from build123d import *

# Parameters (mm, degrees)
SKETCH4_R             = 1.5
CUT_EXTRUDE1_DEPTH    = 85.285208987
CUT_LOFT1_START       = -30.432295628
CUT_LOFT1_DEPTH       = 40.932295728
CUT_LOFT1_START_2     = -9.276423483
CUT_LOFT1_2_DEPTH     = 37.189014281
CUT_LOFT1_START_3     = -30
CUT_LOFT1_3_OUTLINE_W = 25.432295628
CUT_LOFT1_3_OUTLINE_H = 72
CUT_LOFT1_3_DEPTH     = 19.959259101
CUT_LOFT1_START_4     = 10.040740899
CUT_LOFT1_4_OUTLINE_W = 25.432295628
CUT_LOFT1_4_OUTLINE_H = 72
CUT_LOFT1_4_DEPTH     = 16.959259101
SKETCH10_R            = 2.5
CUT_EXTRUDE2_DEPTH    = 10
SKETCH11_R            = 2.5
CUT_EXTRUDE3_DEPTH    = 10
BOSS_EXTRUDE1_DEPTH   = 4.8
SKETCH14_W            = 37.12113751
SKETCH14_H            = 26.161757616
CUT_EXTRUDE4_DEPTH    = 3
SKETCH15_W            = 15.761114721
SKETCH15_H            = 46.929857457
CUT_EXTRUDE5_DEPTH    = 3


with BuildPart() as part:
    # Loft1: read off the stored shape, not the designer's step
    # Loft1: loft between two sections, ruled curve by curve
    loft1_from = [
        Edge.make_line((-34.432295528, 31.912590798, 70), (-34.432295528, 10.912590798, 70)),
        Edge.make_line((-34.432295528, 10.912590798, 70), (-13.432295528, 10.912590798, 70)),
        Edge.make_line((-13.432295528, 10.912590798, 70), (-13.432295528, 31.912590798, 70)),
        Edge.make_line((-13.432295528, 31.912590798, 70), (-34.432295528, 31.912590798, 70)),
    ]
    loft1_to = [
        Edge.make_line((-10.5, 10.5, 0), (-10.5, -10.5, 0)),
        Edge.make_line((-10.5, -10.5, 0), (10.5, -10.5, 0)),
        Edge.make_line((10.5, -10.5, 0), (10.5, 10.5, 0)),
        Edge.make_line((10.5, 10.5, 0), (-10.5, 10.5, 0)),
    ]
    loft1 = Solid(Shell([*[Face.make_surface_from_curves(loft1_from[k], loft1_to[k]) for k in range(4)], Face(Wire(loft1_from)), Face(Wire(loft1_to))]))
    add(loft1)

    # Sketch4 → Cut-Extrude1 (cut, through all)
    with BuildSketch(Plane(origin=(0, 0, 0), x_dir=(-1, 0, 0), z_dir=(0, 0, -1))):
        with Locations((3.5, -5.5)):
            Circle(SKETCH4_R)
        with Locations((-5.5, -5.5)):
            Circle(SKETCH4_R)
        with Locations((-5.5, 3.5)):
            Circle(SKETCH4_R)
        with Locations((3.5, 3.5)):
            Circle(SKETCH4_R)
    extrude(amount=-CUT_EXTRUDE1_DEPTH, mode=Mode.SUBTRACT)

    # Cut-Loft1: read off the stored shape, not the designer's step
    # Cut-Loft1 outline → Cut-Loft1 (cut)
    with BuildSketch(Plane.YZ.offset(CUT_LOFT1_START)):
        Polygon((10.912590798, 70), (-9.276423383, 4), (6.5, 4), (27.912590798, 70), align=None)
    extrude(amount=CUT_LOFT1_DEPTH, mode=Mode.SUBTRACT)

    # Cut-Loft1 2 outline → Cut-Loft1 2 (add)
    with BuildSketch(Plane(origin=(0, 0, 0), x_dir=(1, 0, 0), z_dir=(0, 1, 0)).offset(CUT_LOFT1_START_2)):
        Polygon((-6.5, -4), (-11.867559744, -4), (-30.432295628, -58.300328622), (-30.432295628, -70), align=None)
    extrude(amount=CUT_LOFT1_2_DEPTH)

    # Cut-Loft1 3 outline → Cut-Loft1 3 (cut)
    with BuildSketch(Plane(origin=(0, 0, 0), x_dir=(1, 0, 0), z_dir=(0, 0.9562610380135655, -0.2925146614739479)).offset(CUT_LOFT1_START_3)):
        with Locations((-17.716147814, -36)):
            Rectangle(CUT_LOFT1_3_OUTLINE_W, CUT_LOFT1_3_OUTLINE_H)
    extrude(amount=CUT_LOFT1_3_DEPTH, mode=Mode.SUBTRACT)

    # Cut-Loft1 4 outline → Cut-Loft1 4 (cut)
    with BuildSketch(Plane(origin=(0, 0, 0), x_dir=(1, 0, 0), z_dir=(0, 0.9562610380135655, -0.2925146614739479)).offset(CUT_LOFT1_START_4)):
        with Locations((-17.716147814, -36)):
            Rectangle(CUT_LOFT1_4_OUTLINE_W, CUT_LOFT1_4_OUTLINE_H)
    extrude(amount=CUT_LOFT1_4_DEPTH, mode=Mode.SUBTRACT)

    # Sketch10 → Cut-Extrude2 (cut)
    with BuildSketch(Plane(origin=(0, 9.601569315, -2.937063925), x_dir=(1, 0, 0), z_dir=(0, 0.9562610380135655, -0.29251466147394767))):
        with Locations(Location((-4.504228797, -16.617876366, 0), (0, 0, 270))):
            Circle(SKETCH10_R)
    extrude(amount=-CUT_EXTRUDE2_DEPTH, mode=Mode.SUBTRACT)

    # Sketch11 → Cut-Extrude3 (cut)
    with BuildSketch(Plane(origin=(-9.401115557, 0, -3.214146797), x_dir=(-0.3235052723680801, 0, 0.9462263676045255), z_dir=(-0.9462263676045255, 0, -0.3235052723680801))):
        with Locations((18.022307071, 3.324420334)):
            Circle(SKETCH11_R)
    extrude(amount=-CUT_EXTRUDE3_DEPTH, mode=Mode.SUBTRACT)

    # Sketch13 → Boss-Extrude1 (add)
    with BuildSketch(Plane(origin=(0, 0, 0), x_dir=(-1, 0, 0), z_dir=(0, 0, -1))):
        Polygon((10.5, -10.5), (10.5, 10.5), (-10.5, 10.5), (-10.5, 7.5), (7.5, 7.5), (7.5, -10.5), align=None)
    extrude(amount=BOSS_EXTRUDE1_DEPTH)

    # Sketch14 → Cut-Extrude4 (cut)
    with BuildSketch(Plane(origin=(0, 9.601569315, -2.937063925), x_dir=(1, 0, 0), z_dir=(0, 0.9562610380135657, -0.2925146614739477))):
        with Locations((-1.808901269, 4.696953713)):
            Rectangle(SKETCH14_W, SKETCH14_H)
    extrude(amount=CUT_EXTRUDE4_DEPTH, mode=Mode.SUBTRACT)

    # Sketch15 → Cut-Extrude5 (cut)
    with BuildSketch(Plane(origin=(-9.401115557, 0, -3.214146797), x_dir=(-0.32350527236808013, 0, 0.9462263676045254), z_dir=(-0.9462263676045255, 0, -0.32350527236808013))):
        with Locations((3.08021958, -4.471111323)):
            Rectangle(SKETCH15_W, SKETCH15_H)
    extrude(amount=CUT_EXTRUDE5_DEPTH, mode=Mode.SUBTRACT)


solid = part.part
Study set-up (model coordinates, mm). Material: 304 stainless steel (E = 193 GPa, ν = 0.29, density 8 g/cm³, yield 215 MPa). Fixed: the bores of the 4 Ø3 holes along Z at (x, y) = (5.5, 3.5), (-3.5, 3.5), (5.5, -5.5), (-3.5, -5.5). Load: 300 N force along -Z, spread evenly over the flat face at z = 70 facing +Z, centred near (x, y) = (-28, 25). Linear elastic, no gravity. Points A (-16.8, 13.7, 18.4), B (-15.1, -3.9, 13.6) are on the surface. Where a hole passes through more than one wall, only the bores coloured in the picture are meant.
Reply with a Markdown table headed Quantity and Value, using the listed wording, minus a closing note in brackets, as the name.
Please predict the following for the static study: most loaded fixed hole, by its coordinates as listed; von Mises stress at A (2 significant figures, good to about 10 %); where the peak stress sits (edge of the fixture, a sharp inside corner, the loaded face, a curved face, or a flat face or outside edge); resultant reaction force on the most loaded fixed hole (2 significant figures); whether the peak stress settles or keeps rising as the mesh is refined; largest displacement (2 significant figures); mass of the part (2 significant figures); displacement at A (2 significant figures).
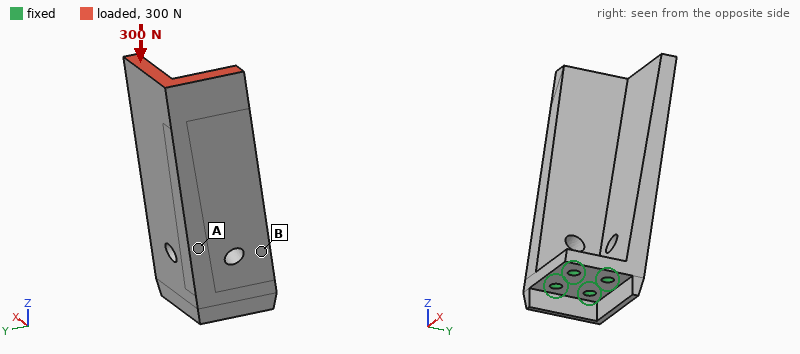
| Quantity | Value |
|---|---|
| most loaded fixed hole, by its coordinates as listed | (-3.5, 3.5) |
| von Mises stress at A | 25 MPa |
| where the peak stress sits | edge of the fixture |
| resultant reaction force on the most loaded fixed hole | 1.3 kN |
| whether the peak stress settles or keeps rising as the mesh is refined | keeps rising |
| largest displacement | 89 µm |
| mass of the part | 110 g |
| displacement at A | 19 µm |
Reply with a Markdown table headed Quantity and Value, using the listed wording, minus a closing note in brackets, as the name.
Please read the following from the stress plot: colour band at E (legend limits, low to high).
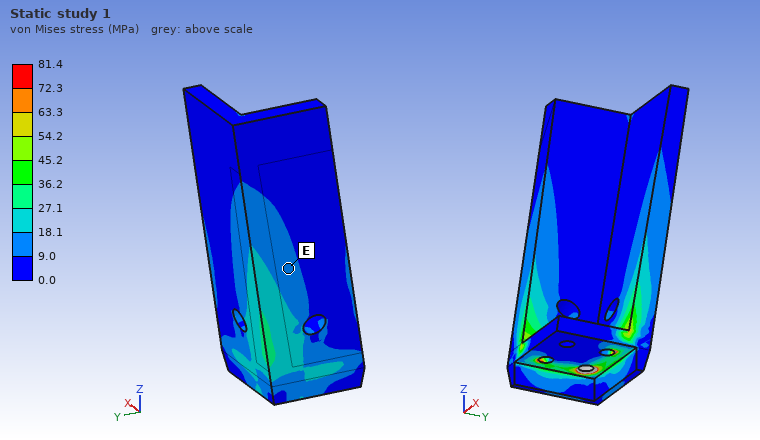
| Quantity | Value |
|---|---|
| colour band at E | 9.0 to 18.1 MPa |
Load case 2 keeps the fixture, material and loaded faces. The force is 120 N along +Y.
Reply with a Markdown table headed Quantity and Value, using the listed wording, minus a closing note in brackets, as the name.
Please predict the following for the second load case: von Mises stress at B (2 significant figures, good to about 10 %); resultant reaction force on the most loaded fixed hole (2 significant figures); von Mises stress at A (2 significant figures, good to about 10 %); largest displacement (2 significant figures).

| Quantity | Value |
|---|---|
| von Mises stress at B | 12 MPa |
| resultant reaction force on the most loaded fixed hole | 650 N |
| von Mises stress at A | 13 MPa |
| largest displacement | 59 µm |
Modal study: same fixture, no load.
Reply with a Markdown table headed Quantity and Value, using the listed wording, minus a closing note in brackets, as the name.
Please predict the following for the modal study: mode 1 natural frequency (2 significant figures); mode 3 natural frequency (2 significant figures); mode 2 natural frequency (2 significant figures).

| Quantity | Value |
|---|---|
| mode 1 natural frequency | 1300 Hz |
| mode 3 natural frequency | 4000 Hz |
| mode 2 natural frequency | 1900 Hz |
